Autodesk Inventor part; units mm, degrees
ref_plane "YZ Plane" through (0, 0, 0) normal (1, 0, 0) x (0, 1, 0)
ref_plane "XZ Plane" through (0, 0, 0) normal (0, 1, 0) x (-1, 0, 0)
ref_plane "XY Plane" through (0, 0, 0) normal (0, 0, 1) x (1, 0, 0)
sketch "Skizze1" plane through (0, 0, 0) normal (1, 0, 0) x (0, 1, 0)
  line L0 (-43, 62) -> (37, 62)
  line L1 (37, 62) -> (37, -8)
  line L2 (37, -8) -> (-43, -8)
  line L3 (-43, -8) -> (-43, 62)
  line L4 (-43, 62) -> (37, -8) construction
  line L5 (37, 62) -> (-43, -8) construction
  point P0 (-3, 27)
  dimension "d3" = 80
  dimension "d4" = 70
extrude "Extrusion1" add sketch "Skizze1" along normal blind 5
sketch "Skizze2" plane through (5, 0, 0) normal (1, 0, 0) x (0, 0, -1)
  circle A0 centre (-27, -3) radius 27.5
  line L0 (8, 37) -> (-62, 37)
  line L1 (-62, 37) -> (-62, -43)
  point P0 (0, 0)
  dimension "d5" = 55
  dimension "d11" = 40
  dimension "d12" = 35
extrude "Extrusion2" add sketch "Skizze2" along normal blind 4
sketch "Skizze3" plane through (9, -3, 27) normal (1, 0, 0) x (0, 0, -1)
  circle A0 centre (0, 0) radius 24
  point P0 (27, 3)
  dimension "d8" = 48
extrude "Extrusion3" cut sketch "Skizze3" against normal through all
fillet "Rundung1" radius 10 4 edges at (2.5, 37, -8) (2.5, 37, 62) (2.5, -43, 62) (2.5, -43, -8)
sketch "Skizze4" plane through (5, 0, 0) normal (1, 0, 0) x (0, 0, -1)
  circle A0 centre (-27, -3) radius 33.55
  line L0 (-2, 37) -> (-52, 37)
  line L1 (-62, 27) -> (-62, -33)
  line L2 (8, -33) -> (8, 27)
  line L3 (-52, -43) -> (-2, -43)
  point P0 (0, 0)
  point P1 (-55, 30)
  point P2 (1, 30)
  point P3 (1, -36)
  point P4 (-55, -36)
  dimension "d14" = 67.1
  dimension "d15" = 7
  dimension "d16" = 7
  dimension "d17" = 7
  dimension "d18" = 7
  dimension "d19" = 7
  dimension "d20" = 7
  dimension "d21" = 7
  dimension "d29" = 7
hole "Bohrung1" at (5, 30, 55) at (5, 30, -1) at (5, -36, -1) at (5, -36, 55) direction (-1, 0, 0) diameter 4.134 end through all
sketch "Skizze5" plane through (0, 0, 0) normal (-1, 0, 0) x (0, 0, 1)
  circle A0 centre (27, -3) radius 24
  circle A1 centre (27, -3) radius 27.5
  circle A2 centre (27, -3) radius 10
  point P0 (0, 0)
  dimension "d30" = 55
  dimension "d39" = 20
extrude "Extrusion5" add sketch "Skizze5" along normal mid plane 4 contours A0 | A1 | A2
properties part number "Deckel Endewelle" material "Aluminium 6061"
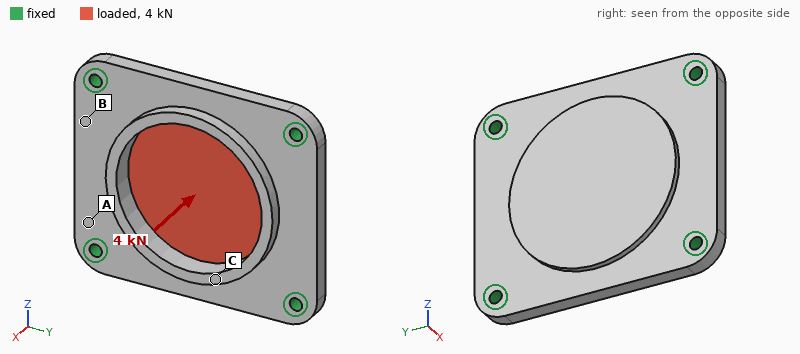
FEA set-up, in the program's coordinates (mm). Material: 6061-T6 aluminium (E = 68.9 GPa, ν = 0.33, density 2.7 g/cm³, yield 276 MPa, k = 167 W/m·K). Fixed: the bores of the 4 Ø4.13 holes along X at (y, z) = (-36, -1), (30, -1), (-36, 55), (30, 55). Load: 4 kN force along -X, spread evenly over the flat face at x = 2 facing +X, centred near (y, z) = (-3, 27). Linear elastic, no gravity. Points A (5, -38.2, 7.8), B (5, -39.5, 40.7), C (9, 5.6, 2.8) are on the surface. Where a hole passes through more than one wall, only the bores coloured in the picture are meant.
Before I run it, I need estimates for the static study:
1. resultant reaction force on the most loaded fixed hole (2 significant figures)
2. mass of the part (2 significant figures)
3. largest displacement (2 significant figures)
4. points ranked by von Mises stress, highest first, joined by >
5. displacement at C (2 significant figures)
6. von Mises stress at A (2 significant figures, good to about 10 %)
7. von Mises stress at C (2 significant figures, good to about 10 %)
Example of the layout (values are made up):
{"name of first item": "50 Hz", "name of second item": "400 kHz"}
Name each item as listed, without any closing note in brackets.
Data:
{"resultant reaction force on the most loaded fixed hole": "1.4 kN", "mass of the part": "78 g", "largest displacement": "0.14 mm", "points ranked by von Mises stress, highest first, joined by >": "C > A > B", "displacement at C": "0.075 mm", "von Mises stress at A": "40 MPa", "von Mises stress at C": "67 MPa"}
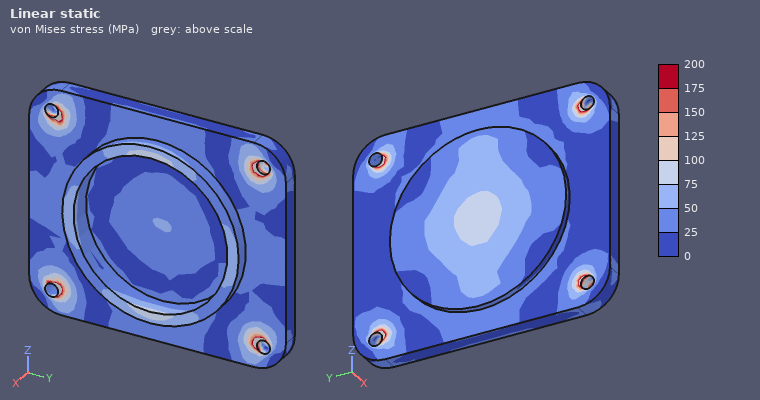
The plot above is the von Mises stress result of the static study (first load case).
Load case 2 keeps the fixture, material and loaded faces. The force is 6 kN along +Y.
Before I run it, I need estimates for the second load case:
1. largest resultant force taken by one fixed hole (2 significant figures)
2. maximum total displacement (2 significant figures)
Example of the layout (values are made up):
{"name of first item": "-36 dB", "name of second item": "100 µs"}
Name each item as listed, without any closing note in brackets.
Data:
{"largest resultant force taken by one fixed hole": "1.6 kN", "maximum total displacement": "15 µm"}
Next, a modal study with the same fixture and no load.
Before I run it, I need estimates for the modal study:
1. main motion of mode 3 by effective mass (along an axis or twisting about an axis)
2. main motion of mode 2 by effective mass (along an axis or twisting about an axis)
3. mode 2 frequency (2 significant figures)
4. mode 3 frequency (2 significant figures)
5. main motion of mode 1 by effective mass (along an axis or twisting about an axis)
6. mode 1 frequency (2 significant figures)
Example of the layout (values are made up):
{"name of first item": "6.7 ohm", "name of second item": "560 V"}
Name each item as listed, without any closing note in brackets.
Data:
{"main motion of mode 3 by effective mass": "twisting about Z", "main motion of mode 2 by effective mass": "twisting about Y", "mode 2 frequency": "7000 Hz", "mode 3 frequency": "8400 Hz", "main motion of mode 1 by effective mass": "along X", "mode 1 frequency": "5200 Hz"}
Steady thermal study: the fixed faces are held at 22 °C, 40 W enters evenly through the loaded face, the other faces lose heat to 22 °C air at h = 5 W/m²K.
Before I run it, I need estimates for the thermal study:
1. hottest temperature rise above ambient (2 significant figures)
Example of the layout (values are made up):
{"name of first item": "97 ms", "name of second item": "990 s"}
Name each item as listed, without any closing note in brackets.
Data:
{"hottest temperature rise above ambient": "15 K"}
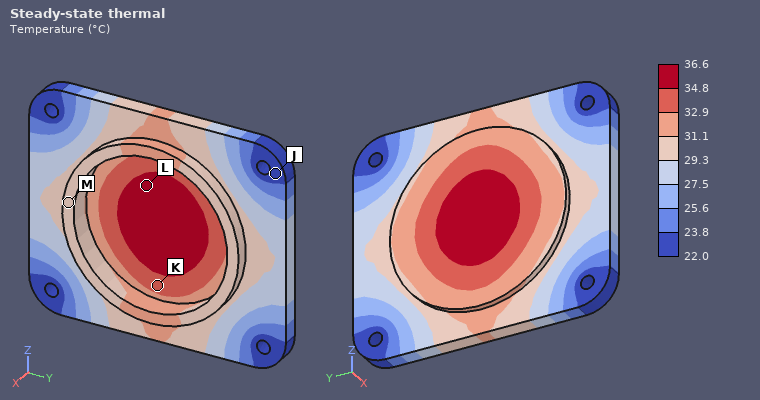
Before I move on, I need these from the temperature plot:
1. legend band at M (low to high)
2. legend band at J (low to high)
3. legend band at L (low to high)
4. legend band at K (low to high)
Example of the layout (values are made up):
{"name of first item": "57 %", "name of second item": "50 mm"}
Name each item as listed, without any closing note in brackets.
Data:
{"legend band at M": "29.3 to 31.1 °C", "legend band at J": "22.0 to 23.8 °C", "legend band at L": "34.8 to 36.6 °C", "legend band at K": "32.9 to 34.8 °C"}
